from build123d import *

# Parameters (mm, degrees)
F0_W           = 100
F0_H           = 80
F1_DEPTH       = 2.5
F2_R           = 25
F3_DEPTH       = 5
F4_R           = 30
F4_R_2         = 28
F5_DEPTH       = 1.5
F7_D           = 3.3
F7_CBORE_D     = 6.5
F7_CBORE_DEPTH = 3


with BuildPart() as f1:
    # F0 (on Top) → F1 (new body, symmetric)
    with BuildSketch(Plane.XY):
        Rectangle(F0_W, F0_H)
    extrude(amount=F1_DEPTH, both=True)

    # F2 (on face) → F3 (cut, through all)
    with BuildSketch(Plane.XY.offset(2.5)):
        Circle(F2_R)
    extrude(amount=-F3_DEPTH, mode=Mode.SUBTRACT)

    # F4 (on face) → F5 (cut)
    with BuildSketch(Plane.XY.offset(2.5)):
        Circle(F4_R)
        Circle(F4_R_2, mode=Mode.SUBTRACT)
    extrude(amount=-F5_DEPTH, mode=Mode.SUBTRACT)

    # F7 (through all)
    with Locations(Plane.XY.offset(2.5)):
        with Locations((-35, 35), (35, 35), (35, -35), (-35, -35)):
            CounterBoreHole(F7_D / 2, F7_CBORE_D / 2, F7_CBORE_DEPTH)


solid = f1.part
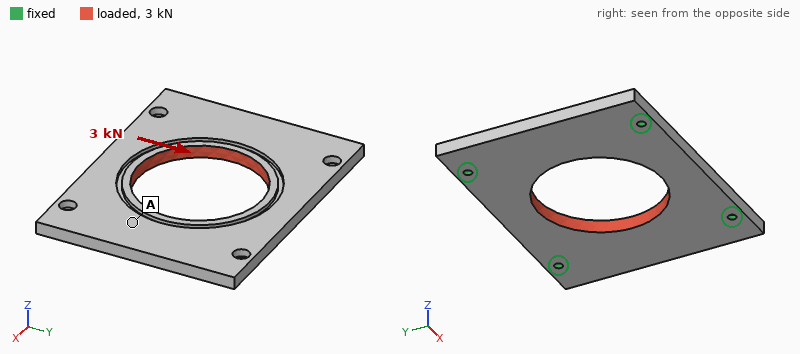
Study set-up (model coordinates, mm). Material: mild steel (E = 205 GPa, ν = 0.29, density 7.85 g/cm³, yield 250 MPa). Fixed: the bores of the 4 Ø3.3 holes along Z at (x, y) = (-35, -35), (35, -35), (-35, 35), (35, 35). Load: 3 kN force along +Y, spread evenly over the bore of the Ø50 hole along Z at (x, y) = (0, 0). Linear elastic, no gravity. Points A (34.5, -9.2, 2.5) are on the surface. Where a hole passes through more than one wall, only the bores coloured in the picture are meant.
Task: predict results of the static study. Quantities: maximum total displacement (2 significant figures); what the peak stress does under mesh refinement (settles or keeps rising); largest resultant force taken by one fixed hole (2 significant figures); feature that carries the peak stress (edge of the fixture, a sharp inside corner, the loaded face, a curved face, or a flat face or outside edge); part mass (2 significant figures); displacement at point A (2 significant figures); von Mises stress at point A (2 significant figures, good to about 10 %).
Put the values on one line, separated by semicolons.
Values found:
4.3 µm; keeps rising; 770 N; edge of the fixture; 230 g; 1.4 µm; 5.3 MPa
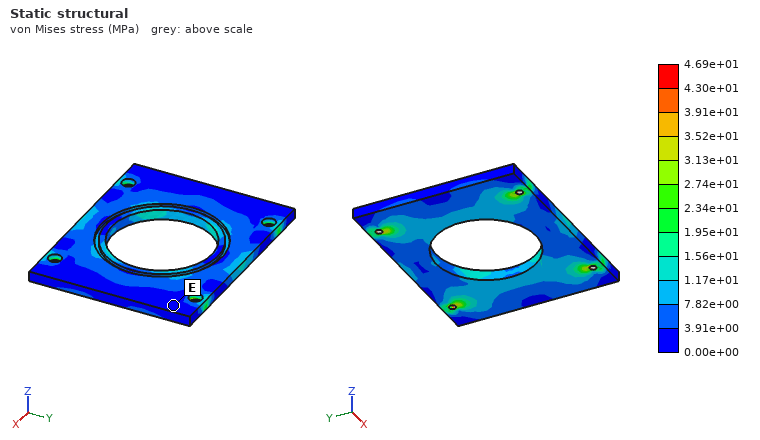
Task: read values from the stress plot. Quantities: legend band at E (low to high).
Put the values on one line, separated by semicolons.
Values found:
0.00e+00 to 3.91e+00 MPa
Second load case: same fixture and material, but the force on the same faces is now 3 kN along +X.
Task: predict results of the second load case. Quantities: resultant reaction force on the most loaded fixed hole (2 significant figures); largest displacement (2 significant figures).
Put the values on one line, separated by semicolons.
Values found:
750 N; 3.8 µm
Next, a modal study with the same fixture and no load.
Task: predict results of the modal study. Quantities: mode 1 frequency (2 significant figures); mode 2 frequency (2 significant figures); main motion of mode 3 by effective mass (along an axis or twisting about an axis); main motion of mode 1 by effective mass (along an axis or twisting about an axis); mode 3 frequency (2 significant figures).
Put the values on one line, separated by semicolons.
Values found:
3300 Hz; 3500 Hz; twisting about Y; along Z; 3700 Hz
